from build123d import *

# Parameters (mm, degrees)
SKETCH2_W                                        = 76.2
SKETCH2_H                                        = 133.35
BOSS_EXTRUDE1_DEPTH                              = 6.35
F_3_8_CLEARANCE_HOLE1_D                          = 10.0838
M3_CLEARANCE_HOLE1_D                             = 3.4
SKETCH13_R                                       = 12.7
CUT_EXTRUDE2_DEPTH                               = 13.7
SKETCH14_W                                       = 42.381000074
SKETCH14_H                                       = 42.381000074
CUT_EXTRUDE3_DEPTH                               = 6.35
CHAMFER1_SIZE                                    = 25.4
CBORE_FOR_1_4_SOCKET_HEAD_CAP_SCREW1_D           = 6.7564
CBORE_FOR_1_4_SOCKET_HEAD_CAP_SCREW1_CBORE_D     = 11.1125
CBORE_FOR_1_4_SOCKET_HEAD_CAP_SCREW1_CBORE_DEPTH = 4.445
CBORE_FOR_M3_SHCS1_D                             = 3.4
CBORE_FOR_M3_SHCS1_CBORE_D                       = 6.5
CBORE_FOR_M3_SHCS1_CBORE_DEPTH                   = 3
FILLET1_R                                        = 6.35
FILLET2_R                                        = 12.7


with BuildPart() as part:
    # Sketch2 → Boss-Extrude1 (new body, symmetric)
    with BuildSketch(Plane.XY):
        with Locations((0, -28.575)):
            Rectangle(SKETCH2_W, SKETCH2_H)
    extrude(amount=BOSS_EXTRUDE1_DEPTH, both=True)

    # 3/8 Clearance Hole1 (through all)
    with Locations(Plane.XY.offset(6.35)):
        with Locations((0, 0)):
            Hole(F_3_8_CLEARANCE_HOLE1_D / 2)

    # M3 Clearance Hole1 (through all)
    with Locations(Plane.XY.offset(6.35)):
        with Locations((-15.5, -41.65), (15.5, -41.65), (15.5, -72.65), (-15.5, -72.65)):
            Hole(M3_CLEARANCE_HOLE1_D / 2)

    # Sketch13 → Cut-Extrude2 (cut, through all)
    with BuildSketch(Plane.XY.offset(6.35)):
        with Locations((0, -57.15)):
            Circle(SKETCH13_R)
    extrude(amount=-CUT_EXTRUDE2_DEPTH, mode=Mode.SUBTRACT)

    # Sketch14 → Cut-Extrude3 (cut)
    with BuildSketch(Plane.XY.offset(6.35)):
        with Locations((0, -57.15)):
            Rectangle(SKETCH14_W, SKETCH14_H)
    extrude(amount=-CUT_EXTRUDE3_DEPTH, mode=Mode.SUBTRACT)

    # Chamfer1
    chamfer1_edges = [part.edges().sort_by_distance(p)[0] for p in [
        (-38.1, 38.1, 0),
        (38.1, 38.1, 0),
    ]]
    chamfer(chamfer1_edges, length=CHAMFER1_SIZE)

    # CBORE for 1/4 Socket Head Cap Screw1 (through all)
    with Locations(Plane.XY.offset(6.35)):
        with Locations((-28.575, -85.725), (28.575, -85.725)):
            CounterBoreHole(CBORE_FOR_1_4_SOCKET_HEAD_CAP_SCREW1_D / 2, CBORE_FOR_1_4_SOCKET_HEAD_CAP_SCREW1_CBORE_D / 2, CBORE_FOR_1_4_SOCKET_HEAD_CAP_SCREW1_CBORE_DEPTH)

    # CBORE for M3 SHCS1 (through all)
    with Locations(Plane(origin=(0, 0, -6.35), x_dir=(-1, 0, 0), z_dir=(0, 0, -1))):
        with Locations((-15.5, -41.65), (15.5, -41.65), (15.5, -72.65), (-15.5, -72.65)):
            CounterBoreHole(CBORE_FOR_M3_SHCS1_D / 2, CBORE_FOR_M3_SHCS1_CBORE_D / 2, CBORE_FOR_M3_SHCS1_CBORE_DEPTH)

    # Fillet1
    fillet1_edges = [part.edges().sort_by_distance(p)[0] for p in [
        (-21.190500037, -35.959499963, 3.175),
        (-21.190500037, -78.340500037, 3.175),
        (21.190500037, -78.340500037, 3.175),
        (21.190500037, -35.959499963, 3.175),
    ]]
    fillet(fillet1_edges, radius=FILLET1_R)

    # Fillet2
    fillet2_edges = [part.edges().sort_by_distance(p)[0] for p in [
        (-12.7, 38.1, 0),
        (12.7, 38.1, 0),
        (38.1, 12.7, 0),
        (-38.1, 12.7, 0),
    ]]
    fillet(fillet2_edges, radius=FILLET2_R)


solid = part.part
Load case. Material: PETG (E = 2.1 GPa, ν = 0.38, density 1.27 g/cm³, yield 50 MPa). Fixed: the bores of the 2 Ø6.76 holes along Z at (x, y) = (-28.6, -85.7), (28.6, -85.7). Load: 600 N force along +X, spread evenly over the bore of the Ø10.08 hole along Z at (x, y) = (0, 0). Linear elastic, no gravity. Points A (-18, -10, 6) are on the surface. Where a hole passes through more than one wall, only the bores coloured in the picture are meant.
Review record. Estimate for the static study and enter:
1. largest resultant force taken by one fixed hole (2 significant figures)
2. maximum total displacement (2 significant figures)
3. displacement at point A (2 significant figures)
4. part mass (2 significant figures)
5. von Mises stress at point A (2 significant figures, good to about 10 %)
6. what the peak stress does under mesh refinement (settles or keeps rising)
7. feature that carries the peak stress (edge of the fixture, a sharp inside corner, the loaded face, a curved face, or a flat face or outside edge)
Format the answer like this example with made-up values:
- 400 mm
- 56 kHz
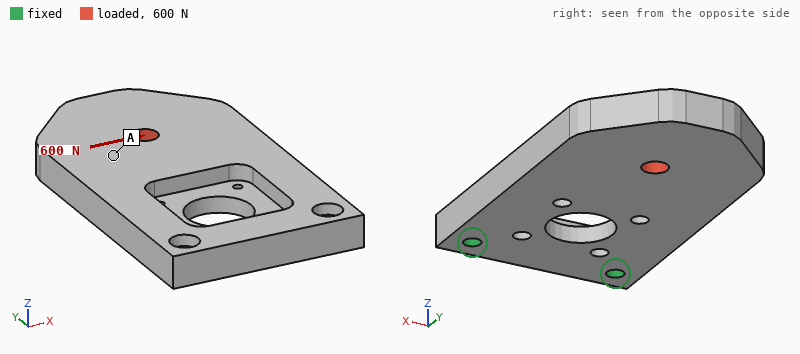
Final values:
- 890 N
- 0.48 mm
- 0.34 mm
- 130 g
- 1.5 MPa
- keeps rising
- edge of the fixture
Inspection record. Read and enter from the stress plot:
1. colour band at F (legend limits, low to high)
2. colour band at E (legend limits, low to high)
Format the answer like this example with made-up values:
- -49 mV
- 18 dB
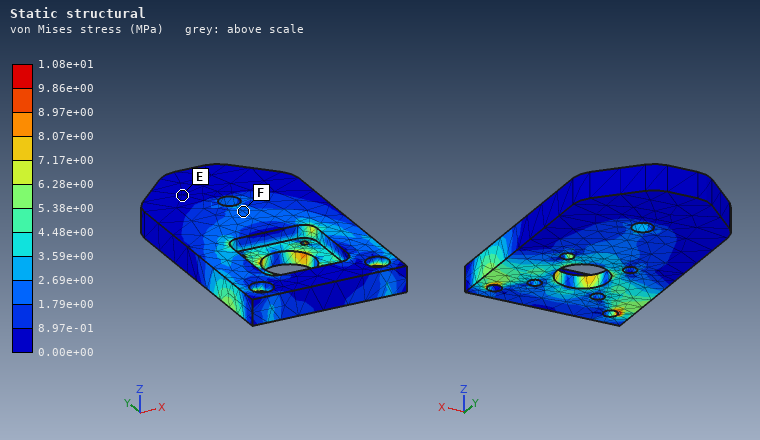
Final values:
- 1.79e+00 to 2.69e+00 MPa
- 0.00e+00 to 8.97e-01 MPa
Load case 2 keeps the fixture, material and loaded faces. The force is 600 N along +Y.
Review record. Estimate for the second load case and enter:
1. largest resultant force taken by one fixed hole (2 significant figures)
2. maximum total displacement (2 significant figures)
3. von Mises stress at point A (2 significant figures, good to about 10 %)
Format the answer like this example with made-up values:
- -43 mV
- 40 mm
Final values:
- 300 N
- 0.28 mm
- 0.69 MPa
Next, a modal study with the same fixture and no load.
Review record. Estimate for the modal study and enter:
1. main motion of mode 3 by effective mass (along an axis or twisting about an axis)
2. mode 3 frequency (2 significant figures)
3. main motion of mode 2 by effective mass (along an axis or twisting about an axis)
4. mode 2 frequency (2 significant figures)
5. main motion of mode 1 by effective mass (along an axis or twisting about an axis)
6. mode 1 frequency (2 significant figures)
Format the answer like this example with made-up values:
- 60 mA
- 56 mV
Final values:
- along X
- 720 Hz
- twisting about Y
- 530 Hz
- along Z
- 130 Hz
